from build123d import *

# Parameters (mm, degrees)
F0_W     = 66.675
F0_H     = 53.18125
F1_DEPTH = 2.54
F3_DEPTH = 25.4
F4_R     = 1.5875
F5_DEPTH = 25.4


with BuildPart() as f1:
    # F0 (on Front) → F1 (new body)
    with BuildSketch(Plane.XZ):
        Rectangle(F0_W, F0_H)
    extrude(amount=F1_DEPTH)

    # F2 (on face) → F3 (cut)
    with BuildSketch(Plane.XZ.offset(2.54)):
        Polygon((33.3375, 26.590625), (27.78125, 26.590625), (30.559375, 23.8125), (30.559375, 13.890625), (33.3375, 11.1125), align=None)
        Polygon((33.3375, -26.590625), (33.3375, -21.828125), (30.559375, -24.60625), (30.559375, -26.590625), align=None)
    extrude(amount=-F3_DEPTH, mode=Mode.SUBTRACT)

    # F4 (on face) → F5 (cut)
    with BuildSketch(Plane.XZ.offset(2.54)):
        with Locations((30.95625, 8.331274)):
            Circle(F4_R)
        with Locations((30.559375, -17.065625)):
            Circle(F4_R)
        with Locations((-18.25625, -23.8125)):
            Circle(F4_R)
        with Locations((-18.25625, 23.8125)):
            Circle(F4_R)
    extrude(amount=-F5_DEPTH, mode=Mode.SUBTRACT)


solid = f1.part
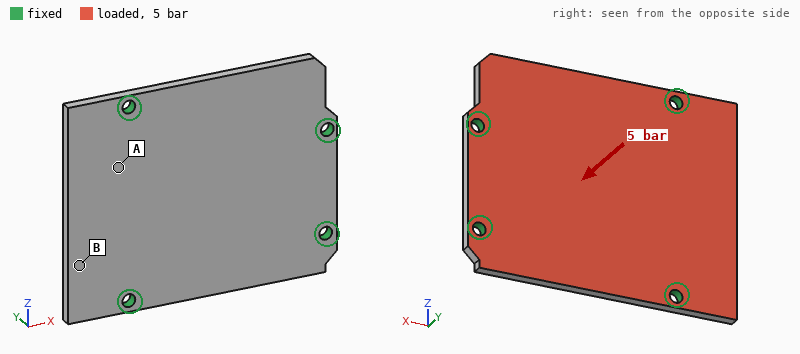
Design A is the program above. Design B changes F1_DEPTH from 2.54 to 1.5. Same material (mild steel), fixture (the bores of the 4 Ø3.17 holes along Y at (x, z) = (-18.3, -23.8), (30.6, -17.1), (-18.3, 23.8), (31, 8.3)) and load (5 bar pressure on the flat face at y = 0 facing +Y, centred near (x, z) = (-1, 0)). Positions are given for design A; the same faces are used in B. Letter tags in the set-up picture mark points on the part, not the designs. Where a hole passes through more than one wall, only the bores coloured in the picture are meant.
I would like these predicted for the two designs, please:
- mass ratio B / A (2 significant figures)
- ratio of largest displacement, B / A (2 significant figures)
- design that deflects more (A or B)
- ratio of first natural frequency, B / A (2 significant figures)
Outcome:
0.59
4.6
B
0.61
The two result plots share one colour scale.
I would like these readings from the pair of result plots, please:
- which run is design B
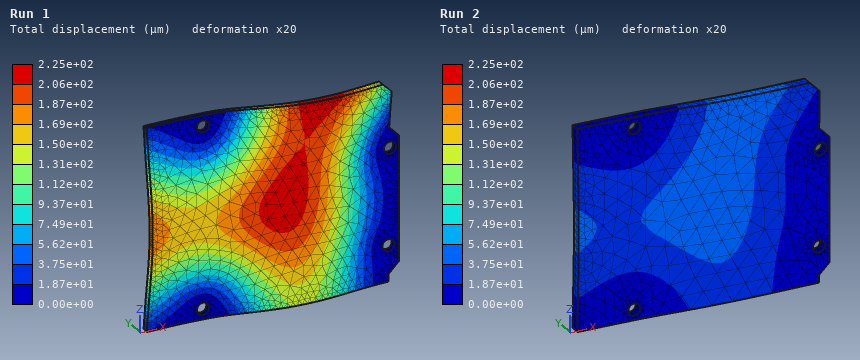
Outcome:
Run 1
